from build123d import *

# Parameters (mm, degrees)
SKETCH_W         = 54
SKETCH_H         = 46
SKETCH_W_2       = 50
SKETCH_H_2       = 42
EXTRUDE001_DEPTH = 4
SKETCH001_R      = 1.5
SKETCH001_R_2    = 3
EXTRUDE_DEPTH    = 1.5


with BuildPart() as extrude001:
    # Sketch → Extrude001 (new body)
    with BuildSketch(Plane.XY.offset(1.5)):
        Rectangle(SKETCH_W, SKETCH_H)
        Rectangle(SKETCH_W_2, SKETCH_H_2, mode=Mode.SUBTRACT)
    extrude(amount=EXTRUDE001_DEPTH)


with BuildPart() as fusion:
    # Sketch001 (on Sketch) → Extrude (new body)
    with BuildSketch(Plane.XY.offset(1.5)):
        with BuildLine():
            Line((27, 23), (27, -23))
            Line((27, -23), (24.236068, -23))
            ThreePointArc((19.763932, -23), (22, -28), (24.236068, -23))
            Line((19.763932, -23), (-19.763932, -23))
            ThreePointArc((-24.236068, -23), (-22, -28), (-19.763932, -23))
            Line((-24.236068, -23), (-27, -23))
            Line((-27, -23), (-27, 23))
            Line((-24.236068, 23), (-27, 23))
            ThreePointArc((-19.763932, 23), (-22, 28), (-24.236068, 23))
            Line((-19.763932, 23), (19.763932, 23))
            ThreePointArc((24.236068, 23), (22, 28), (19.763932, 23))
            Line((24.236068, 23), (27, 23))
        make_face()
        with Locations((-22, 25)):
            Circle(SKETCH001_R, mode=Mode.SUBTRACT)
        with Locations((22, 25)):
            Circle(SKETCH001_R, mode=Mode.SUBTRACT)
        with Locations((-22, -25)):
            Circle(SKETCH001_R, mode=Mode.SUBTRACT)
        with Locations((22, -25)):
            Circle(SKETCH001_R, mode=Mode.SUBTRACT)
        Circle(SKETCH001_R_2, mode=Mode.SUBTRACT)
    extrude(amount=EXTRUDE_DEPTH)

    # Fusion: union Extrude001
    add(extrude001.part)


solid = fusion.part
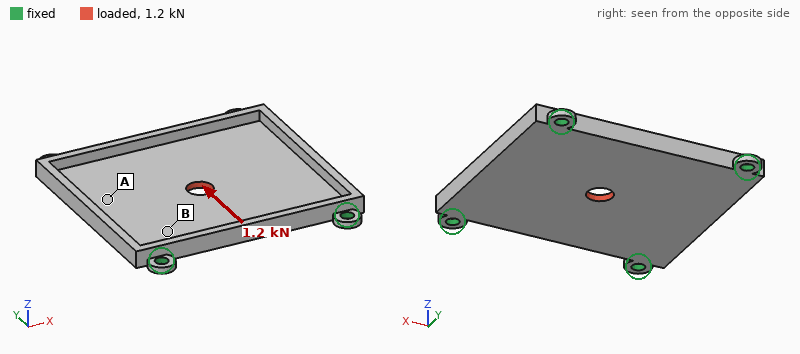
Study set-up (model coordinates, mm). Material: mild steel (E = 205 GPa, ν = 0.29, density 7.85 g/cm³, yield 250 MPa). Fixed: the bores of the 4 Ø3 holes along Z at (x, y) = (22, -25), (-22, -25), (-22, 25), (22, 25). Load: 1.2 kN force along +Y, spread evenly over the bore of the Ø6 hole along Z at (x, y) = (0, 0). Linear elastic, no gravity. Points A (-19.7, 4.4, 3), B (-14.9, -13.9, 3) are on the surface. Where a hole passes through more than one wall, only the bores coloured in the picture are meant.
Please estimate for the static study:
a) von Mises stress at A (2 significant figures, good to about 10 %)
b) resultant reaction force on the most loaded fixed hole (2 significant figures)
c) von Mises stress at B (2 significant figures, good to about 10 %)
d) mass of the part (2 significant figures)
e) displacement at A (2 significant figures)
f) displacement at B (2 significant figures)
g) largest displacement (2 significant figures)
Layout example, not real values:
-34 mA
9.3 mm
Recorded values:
11 MPa
320 N
21 MPa
37 g
1.5 µm
1.9 µm
4.6 µm
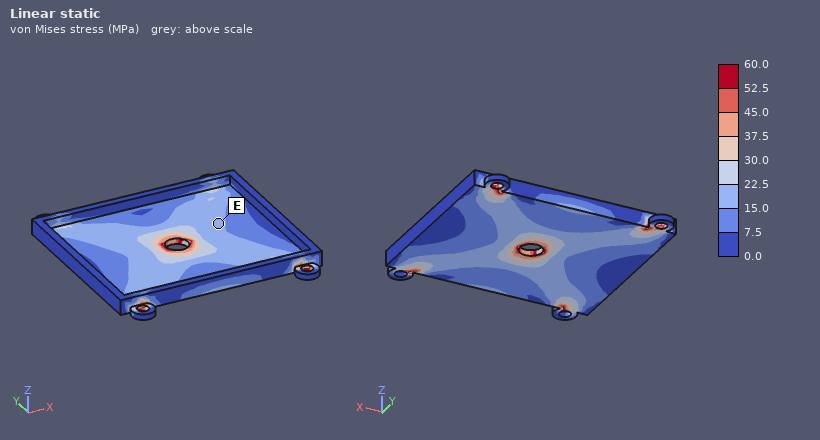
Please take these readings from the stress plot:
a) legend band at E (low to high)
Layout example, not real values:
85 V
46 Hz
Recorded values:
15.0 to 22.5 MPa
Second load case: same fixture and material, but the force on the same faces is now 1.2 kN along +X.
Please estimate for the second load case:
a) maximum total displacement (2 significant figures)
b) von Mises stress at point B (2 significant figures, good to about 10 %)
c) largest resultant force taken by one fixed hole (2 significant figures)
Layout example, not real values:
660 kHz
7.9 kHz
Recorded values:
5.8 µm
21 MPa
320 N
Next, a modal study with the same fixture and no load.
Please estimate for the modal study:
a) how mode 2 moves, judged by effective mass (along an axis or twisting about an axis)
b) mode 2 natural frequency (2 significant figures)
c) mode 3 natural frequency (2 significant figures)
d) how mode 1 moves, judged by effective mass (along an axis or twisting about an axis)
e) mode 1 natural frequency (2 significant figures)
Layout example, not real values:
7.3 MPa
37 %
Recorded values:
twisting about Y
4800 Hz
5800 Hz
along Z
2800 Hz
